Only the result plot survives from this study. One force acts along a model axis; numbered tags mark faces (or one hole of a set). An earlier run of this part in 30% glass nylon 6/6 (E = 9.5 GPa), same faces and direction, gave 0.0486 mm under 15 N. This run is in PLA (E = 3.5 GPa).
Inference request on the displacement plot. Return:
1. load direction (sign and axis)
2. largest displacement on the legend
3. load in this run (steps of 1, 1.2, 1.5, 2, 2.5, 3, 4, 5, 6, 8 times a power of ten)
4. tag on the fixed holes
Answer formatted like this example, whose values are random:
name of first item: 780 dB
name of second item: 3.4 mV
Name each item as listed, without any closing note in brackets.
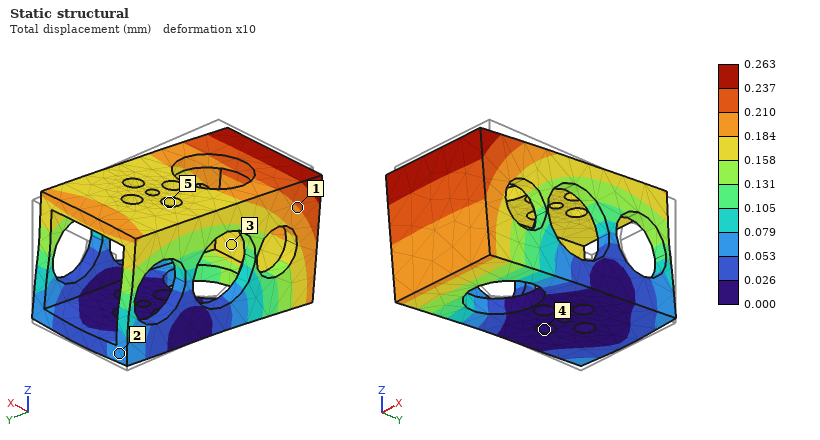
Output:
load direction: -Y
largest displacement on the legend: 0.263 mm
load in this run: 30 N
tag on the fixed holes: 4
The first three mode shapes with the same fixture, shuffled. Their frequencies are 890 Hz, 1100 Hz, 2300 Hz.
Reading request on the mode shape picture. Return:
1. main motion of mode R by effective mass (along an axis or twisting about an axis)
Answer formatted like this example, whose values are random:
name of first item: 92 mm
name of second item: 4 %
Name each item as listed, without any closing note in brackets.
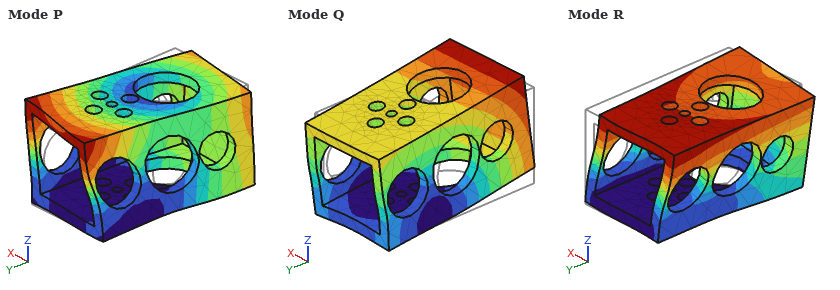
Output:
main motion of mode R by effective mass: along X
